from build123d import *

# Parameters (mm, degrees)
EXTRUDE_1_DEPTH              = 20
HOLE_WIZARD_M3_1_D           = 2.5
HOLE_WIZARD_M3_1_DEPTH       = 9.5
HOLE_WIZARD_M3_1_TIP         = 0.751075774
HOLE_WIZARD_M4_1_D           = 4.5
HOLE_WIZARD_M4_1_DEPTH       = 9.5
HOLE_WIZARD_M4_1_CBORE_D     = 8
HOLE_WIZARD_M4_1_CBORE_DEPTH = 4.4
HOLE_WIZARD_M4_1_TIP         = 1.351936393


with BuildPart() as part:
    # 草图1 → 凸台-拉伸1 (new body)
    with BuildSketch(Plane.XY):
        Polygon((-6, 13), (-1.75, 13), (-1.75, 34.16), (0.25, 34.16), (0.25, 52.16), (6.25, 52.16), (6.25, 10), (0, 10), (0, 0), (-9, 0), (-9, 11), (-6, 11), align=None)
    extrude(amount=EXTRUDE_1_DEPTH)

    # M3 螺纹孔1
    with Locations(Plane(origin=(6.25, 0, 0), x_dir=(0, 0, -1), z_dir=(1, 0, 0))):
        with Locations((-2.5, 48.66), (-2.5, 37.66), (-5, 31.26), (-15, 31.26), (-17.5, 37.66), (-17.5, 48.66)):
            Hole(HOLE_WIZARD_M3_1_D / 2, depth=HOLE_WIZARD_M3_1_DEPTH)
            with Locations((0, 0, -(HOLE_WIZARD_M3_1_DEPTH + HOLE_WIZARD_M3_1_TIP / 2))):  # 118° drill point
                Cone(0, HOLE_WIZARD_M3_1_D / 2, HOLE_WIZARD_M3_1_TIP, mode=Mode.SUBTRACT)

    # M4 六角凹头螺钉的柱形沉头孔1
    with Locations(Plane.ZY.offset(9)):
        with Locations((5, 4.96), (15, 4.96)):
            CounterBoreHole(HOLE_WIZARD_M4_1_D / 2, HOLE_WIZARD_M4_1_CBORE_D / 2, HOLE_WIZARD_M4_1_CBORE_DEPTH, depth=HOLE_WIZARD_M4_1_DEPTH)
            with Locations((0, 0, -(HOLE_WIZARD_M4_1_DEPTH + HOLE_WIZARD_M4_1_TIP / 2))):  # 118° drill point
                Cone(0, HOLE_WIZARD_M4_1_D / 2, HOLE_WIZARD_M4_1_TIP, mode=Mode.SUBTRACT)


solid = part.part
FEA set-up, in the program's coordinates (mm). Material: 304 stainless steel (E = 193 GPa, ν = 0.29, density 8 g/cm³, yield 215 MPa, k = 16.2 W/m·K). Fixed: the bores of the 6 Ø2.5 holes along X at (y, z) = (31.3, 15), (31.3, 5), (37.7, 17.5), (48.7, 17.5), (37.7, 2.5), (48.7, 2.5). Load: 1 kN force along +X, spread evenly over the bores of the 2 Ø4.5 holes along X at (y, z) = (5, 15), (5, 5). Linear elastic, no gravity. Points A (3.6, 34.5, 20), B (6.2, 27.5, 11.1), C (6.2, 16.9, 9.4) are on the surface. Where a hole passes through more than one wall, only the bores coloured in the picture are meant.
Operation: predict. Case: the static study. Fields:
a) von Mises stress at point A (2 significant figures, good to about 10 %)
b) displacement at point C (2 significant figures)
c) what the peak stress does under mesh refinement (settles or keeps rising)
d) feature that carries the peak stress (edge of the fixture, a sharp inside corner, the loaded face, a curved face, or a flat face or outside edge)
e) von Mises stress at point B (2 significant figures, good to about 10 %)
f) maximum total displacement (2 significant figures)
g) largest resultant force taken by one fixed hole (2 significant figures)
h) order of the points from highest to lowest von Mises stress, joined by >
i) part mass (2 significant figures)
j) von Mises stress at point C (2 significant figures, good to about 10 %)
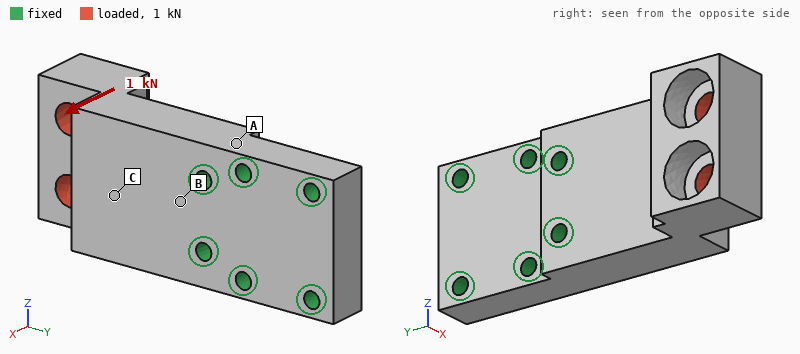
25 MPa
17 µm
keeps rising
edge of the fixture
85 MPa
72 µm
790 N
B > C > A
59 g
52 MPa
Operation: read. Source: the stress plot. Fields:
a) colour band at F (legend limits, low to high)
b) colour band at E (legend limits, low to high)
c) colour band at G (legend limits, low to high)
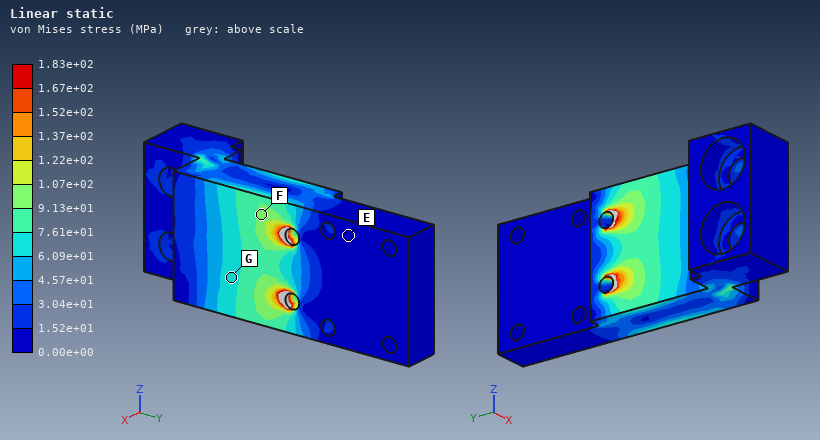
9.13e+01 to 1.07e+02 MPa
0.00e+00 to 1.52e+01 MPa
6.09e+01 to 7.61e+01 MPa
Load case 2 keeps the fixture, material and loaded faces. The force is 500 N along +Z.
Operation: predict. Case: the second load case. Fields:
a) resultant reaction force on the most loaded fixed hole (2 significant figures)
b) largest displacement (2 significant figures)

860 N
8.5 µm
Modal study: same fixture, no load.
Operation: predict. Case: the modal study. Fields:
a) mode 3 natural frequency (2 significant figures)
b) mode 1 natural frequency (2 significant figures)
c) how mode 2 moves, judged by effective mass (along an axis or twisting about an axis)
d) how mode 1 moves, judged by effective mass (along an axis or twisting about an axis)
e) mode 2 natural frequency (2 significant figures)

16 kHz
5900 Hz
along Z
along X
11 kHz
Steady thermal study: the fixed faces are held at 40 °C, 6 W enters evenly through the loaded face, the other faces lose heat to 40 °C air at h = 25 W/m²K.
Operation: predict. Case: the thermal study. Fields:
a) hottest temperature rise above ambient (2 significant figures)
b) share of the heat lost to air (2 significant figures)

63 K
33 %
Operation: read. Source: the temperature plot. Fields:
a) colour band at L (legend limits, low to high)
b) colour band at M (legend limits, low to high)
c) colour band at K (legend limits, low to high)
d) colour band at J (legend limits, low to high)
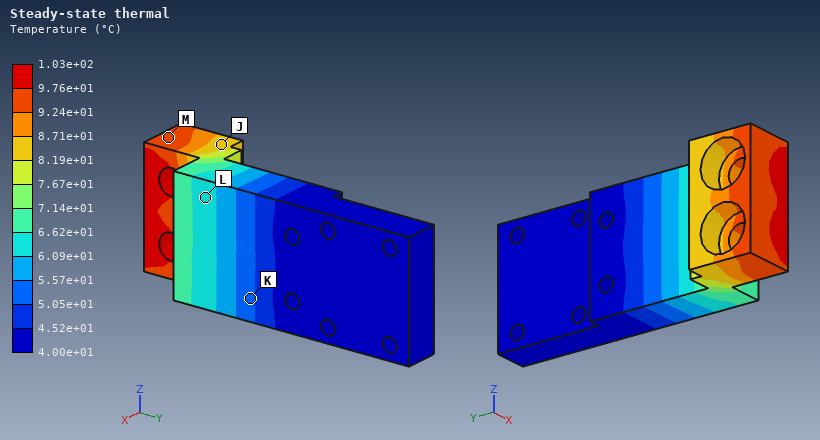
6.09e+01 to 6.62e+01 °C
9.24e+01 to 9.76e+01 °C
5.05e+01 to 5.57e+01 °C
8.19e+01 to 8.71e+01 °C
